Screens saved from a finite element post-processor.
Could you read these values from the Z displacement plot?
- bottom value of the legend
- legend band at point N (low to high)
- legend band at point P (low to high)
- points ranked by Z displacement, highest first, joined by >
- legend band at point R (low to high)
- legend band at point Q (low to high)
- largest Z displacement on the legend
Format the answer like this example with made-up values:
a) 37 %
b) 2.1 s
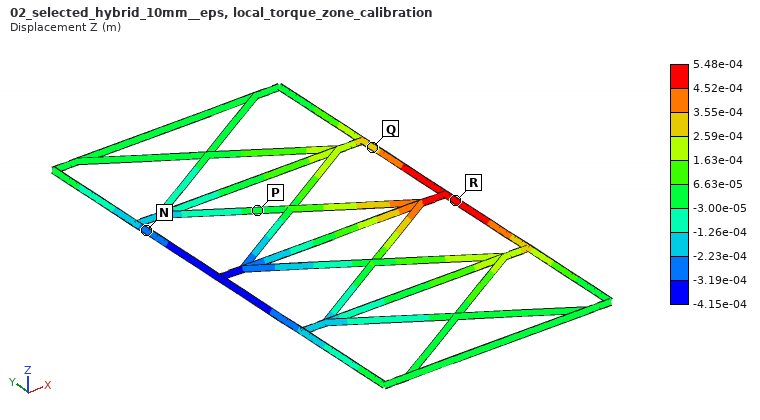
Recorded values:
a) -4.15e-04 m
b) -3.19e-04 to -2.23e-04 m
c) -3.00e-05 to 6.63e-05 m
d) R > Q > P > N
e) 4.52e-04 to 5.48e-04 m
f) 2.59e-04 to 3.55e-04 m
g) 5.48e-04 m
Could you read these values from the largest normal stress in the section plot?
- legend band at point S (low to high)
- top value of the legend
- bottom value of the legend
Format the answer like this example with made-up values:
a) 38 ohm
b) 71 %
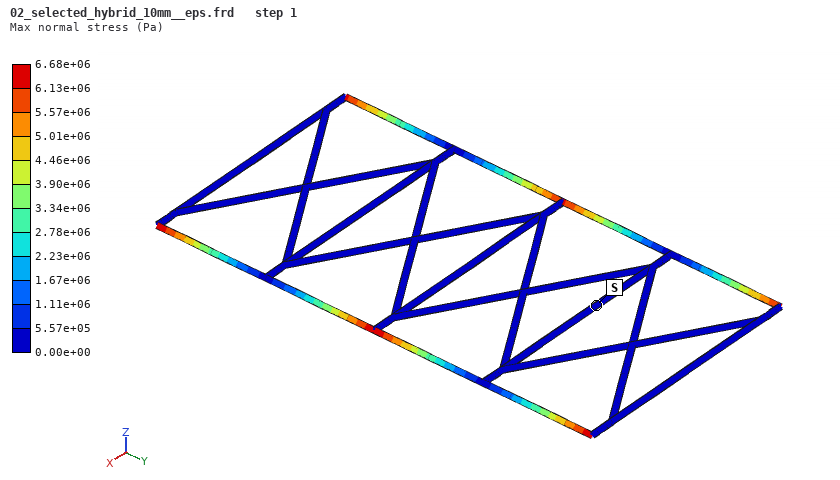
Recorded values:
a) 0.00e+00 to 5.57e+05 Pa
b) 6.68e+06 Pa
c) 0.00e+00 Pa
